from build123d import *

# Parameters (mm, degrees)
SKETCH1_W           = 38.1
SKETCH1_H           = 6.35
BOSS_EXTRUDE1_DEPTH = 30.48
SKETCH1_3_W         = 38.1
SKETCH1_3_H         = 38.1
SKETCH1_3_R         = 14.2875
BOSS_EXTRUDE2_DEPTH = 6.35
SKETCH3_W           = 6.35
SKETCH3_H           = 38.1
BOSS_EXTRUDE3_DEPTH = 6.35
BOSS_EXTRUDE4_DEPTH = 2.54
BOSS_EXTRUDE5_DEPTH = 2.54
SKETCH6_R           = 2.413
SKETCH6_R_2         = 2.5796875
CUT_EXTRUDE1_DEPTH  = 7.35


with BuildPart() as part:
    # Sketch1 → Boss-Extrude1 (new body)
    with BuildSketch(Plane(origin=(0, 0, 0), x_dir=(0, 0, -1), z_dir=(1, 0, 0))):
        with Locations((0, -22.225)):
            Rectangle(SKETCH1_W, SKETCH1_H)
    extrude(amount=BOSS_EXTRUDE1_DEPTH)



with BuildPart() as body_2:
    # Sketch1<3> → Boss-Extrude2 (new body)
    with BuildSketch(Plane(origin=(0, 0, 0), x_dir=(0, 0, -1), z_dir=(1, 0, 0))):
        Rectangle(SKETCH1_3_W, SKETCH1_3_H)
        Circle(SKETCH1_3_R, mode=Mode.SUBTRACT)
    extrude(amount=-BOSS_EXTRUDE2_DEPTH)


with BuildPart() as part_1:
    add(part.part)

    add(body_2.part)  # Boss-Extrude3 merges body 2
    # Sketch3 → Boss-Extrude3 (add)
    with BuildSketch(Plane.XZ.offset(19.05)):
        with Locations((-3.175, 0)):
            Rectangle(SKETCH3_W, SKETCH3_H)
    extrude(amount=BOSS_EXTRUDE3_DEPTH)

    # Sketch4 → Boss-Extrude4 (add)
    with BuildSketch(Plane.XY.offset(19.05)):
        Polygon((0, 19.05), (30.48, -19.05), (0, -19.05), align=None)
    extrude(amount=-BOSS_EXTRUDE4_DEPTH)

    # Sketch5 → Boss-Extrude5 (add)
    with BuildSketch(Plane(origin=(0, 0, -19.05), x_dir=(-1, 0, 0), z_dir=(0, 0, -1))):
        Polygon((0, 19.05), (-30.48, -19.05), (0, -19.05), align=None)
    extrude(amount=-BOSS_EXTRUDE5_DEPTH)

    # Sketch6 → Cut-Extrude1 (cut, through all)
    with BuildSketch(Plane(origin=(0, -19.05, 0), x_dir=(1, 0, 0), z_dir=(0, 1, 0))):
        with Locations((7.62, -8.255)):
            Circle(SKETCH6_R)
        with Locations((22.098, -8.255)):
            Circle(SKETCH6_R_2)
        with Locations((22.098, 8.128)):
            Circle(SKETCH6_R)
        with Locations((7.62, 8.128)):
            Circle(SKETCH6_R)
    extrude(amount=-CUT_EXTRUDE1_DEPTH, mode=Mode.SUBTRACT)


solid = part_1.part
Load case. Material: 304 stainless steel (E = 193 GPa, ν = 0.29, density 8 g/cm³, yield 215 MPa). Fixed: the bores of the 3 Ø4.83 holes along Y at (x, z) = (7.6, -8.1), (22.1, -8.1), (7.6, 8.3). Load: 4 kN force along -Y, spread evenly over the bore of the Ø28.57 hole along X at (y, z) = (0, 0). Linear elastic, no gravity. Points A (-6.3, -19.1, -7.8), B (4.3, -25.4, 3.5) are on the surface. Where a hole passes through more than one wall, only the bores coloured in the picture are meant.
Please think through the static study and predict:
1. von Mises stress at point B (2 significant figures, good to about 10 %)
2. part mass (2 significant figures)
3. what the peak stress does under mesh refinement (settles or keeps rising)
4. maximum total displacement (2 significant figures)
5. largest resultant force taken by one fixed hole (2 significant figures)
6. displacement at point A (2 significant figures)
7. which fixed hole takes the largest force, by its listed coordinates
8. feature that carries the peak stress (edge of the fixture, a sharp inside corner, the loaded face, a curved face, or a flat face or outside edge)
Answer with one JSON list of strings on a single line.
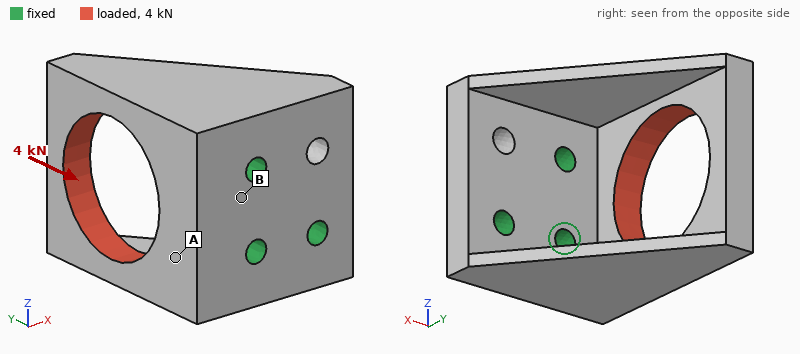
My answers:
["51 MPa", "130 g", "keeps rising", "45 µm", "2.7 kN", "11 µm", "(7.6, -8.1)", "edge of the fixture"]
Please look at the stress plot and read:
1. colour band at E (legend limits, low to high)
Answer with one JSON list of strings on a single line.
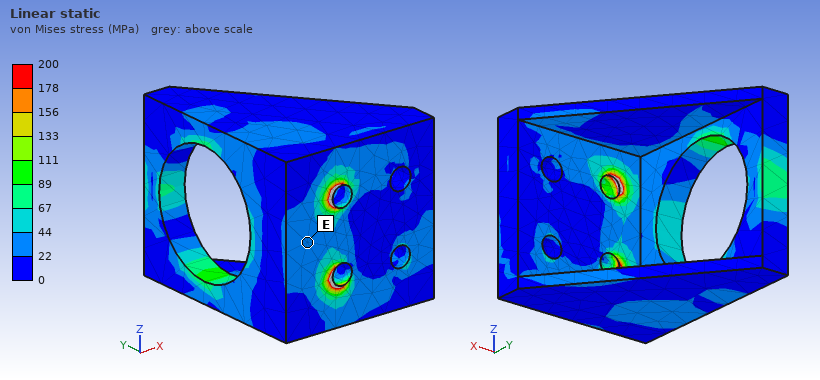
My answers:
["22 to 44 MPa"]
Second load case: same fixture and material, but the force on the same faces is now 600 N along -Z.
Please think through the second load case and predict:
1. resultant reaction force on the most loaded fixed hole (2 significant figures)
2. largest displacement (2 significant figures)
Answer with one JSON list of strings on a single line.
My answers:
["670 N", "19 µm"]
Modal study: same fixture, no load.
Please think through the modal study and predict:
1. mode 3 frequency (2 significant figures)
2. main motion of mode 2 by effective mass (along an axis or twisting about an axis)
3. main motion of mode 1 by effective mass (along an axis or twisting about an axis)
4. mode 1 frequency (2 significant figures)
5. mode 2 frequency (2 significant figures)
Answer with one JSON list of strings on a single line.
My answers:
["8800 Hz", "along X", "along Z", "4200 Hz", "5100 Hz"]
